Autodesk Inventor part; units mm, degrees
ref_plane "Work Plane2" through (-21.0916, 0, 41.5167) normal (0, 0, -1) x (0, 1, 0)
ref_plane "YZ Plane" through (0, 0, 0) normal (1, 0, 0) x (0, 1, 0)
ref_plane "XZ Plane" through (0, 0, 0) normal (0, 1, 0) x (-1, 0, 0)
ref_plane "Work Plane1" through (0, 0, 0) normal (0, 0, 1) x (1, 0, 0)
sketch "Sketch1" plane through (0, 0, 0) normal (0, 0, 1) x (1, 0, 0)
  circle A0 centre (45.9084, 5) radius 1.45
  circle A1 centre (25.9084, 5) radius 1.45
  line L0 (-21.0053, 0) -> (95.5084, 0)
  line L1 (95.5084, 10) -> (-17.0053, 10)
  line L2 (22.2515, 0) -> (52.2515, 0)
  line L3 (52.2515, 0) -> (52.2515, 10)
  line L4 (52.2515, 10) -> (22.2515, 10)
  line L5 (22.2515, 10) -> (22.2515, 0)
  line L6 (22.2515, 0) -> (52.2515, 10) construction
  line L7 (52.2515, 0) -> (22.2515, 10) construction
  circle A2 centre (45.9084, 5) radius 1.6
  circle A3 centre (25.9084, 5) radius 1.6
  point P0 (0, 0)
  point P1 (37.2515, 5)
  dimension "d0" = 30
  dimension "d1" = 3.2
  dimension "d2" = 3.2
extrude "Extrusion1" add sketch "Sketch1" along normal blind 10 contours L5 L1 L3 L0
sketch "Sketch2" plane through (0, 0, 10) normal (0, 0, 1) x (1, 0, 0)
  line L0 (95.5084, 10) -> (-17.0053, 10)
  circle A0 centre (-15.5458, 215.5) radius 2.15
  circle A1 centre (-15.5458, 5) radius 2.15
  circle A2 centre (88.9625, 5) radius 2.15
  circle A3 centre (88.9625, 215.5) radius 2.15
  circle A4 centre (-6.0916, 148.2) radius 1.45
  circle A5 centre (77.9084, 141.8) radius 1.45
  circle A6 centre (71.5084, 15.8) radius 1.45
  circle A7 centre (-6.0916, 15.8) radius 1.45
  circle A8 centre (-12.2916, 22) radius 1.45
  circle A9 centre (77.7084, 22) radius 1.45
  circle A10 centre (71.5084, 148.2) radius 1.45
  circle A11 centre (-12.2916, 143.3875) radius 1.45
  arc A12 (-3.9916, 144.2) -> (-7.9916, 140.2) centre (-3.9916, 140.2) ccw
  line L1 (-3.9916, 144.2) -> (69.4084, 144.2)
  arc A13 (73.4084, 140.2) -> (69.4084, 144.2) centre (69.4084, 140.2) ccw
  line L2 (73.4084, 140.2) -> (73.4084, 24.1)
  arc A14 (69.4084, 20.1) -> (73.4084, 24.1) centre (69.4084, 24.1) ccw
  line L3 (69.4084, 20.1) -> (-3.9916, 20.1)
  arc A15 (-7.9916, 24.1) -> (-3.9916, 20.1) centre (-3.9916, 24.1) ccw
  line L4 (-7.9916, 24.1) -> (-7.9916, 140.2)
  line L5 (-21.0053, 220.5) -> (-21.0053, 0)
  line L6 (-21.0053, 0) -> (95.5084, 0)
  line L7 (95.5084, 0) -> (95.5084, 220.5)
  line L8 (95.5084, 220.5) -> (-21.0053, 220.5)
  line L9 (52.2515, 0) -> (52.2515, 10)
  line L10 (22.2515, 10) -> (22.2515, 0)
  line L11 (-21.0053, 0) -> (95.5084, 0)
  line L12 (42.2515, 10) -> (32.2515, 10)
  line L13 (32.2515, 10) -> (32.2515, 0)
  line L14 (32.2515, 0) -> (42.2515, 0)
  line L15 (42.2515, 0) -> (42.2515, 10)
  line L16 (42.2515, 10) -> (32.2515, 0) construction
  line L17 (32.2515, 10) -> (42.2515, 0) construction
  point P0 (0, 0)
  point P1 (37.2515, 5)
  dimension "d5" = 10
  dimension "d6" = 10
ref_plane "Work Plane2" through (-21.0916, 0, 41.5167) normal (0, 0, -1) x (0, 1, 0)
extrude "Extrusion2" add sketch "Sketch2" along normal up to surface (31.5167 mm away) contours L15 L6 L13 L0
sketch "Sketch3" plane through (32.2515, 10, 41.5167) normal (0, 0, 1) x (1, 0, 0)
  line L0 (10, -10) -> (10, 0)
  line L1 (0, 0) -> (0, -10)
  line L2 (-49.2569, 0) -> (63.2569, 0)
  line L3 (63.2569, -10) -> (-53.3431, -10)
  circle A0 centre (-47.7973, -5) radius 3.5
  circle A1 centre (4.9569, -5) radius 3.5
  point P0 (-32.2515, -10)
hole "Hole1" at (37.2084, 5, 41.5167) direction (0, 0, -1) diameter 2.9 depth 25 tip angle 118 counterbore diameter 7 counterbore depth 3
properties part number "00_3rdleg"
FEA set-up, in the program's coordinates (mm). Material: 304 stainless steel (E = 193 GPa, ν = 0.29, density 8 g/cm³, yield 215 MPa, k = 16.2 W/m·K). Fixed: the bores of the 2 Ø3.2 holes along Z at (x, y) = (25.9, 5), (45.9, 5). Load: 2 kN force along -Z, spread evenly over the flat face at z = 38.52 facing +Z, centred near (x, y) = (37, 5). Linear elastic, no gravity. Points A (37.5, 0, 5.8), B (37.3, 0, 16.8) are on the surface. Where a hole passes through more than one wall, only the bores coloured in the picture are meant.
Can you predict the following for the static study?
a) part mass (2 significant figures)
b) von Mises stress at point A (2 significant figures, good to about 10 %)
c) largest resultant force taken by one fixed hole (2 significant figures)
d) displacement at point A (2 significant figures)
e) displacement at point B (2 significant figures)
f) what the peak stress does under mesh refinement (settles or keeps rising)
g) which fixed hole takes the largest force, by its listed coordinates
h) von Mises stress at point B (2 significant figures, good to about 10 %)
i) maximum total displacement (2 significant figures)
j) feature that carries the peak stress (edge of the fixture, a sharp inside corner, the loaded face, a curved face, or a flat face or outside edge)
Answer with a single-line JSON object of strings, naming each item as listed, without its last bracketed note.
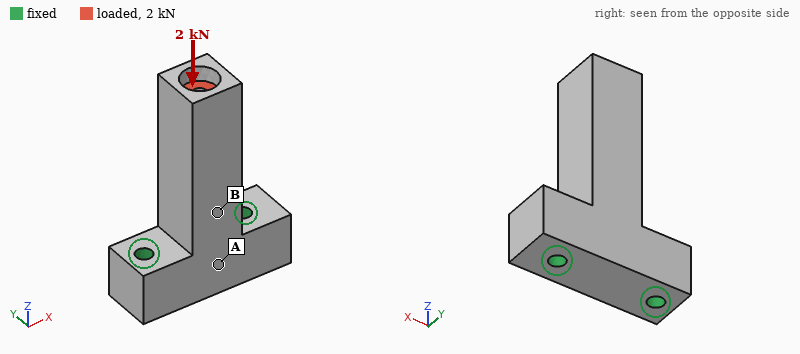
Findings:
{"part mass": "46 g", "von Mises stress at point A": "8.3 MPa", "largest resultant force taken by one fixed hole": "1.2 kN", "displacement at point A": "1.2 µm", "displacement at point B": "2.0 µm", "what the peak stress does under mesh refinement": "keeps rising", "which fixed hole takes the largest force, by its listed coordinates": "(45.9, 5)", "von Mises stress at point B": "21 MPa", "maximum total displacement": "5.3 µm", "feature that carries the peak stress": "edge of the fixture"}
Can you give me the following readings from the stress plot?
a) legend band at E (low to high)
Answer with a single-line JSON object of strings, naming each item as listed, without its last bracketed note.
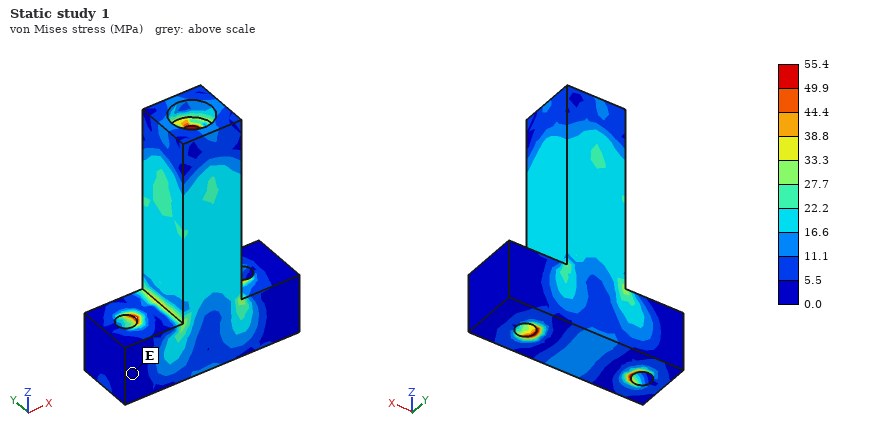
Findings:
{"legend band at E": "0.0 to 5.5 MPa"}
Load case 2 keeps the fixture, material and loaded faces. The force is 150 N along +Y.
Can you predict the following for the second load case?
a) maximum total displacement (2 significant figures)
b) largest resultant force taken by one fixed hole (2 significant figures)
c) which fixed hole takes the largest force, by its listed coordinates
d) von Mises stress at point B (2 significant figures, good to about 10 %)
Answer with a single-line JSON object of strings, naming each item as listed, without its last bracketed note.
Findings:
{"maximum total displacement": "18 µm", "largest resultant force taken by one fixed hole": "93 N", "which fixed hole takes the largest force, by its listed coordinates": "(45.9, 5)", "von Mises stress at point B": "20 MPa"}
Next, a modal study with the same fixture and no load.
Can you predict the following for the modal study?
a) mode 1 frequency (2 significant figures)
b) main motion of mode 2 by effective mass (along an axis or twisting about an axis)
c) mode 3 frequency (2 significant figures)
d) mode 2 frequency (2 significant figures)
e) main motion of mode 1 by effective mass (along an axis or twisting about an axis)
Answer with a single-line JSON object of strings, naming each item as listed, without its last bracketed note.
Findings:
{"mode 1 frequency": "5400 Hz", "main motion of mode 2 by effective mass": "along X", "mode 3 frequency": "21 kHz", "mode 2 frequency": "6700 Hz", "main motion of mode 1 by effective mass": "along Y"}
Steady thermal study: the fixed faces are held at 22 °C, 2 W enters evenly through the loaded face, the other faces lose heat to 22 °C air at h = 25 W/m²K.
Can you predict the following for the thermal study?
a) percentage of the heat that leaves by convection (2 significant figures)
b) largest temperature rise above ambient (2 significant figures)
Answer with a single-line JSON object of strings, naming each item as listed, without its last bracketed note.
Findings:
{"percentage of the heat that leaves by convection": "39 %", "largest temperature rise above ambient": "35 K"}
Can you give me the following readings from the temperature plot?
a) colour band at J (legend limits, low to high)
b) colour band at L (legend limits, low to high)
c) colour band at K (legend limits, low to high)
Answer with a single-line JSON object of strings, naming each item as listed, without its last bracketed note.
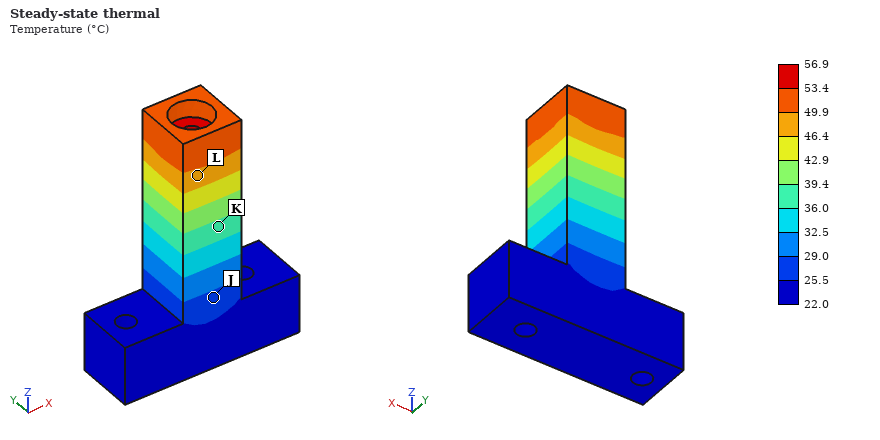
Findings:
{"colour band at J": "25.5 to 29.0 °C", "colour band at L": "46.4 to 49.9 °C", "colour band at K": "36.0 to 39.4 °C"}
